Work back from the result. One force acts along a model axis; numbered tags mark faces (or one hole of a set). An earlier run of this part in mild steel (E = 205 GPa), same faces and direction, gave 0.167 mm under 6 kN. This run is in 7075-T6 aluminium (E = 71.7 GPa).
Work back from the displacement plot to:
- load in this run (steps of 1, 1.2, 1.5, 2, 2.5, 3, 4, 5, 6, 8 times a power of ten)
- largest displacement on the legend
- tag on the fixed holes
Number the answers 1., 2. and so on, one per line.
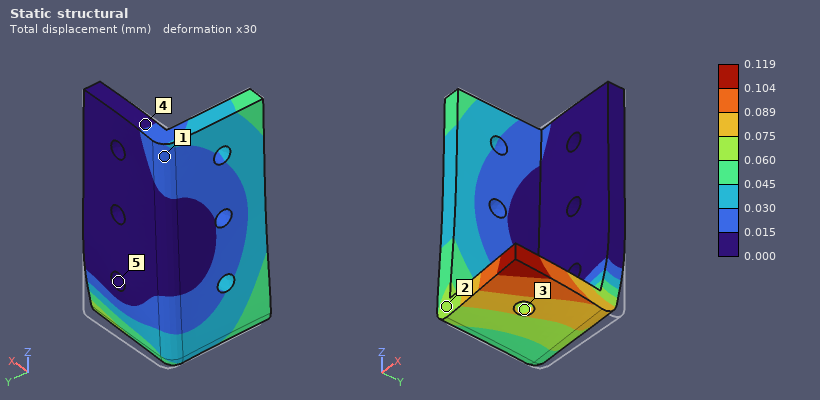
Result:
1. 1.5 kN
2. 0.119 mm
3. 5
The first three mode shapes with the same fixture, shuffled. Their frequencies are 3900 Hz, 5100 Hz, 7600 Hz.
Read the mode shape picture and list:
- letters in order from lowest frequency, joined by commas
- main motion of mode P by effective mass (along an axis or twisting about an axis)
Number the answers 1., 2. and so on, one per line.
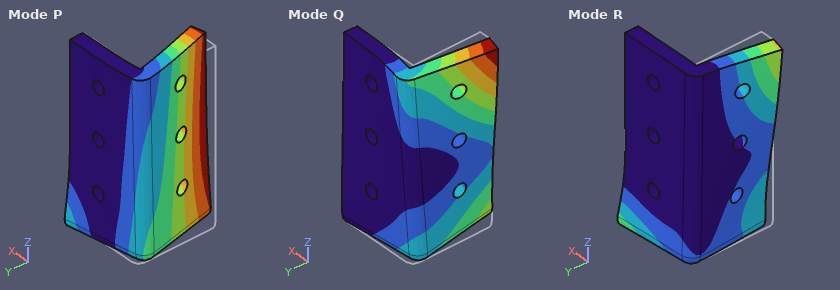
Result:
1. P, Q, R
2. along X
